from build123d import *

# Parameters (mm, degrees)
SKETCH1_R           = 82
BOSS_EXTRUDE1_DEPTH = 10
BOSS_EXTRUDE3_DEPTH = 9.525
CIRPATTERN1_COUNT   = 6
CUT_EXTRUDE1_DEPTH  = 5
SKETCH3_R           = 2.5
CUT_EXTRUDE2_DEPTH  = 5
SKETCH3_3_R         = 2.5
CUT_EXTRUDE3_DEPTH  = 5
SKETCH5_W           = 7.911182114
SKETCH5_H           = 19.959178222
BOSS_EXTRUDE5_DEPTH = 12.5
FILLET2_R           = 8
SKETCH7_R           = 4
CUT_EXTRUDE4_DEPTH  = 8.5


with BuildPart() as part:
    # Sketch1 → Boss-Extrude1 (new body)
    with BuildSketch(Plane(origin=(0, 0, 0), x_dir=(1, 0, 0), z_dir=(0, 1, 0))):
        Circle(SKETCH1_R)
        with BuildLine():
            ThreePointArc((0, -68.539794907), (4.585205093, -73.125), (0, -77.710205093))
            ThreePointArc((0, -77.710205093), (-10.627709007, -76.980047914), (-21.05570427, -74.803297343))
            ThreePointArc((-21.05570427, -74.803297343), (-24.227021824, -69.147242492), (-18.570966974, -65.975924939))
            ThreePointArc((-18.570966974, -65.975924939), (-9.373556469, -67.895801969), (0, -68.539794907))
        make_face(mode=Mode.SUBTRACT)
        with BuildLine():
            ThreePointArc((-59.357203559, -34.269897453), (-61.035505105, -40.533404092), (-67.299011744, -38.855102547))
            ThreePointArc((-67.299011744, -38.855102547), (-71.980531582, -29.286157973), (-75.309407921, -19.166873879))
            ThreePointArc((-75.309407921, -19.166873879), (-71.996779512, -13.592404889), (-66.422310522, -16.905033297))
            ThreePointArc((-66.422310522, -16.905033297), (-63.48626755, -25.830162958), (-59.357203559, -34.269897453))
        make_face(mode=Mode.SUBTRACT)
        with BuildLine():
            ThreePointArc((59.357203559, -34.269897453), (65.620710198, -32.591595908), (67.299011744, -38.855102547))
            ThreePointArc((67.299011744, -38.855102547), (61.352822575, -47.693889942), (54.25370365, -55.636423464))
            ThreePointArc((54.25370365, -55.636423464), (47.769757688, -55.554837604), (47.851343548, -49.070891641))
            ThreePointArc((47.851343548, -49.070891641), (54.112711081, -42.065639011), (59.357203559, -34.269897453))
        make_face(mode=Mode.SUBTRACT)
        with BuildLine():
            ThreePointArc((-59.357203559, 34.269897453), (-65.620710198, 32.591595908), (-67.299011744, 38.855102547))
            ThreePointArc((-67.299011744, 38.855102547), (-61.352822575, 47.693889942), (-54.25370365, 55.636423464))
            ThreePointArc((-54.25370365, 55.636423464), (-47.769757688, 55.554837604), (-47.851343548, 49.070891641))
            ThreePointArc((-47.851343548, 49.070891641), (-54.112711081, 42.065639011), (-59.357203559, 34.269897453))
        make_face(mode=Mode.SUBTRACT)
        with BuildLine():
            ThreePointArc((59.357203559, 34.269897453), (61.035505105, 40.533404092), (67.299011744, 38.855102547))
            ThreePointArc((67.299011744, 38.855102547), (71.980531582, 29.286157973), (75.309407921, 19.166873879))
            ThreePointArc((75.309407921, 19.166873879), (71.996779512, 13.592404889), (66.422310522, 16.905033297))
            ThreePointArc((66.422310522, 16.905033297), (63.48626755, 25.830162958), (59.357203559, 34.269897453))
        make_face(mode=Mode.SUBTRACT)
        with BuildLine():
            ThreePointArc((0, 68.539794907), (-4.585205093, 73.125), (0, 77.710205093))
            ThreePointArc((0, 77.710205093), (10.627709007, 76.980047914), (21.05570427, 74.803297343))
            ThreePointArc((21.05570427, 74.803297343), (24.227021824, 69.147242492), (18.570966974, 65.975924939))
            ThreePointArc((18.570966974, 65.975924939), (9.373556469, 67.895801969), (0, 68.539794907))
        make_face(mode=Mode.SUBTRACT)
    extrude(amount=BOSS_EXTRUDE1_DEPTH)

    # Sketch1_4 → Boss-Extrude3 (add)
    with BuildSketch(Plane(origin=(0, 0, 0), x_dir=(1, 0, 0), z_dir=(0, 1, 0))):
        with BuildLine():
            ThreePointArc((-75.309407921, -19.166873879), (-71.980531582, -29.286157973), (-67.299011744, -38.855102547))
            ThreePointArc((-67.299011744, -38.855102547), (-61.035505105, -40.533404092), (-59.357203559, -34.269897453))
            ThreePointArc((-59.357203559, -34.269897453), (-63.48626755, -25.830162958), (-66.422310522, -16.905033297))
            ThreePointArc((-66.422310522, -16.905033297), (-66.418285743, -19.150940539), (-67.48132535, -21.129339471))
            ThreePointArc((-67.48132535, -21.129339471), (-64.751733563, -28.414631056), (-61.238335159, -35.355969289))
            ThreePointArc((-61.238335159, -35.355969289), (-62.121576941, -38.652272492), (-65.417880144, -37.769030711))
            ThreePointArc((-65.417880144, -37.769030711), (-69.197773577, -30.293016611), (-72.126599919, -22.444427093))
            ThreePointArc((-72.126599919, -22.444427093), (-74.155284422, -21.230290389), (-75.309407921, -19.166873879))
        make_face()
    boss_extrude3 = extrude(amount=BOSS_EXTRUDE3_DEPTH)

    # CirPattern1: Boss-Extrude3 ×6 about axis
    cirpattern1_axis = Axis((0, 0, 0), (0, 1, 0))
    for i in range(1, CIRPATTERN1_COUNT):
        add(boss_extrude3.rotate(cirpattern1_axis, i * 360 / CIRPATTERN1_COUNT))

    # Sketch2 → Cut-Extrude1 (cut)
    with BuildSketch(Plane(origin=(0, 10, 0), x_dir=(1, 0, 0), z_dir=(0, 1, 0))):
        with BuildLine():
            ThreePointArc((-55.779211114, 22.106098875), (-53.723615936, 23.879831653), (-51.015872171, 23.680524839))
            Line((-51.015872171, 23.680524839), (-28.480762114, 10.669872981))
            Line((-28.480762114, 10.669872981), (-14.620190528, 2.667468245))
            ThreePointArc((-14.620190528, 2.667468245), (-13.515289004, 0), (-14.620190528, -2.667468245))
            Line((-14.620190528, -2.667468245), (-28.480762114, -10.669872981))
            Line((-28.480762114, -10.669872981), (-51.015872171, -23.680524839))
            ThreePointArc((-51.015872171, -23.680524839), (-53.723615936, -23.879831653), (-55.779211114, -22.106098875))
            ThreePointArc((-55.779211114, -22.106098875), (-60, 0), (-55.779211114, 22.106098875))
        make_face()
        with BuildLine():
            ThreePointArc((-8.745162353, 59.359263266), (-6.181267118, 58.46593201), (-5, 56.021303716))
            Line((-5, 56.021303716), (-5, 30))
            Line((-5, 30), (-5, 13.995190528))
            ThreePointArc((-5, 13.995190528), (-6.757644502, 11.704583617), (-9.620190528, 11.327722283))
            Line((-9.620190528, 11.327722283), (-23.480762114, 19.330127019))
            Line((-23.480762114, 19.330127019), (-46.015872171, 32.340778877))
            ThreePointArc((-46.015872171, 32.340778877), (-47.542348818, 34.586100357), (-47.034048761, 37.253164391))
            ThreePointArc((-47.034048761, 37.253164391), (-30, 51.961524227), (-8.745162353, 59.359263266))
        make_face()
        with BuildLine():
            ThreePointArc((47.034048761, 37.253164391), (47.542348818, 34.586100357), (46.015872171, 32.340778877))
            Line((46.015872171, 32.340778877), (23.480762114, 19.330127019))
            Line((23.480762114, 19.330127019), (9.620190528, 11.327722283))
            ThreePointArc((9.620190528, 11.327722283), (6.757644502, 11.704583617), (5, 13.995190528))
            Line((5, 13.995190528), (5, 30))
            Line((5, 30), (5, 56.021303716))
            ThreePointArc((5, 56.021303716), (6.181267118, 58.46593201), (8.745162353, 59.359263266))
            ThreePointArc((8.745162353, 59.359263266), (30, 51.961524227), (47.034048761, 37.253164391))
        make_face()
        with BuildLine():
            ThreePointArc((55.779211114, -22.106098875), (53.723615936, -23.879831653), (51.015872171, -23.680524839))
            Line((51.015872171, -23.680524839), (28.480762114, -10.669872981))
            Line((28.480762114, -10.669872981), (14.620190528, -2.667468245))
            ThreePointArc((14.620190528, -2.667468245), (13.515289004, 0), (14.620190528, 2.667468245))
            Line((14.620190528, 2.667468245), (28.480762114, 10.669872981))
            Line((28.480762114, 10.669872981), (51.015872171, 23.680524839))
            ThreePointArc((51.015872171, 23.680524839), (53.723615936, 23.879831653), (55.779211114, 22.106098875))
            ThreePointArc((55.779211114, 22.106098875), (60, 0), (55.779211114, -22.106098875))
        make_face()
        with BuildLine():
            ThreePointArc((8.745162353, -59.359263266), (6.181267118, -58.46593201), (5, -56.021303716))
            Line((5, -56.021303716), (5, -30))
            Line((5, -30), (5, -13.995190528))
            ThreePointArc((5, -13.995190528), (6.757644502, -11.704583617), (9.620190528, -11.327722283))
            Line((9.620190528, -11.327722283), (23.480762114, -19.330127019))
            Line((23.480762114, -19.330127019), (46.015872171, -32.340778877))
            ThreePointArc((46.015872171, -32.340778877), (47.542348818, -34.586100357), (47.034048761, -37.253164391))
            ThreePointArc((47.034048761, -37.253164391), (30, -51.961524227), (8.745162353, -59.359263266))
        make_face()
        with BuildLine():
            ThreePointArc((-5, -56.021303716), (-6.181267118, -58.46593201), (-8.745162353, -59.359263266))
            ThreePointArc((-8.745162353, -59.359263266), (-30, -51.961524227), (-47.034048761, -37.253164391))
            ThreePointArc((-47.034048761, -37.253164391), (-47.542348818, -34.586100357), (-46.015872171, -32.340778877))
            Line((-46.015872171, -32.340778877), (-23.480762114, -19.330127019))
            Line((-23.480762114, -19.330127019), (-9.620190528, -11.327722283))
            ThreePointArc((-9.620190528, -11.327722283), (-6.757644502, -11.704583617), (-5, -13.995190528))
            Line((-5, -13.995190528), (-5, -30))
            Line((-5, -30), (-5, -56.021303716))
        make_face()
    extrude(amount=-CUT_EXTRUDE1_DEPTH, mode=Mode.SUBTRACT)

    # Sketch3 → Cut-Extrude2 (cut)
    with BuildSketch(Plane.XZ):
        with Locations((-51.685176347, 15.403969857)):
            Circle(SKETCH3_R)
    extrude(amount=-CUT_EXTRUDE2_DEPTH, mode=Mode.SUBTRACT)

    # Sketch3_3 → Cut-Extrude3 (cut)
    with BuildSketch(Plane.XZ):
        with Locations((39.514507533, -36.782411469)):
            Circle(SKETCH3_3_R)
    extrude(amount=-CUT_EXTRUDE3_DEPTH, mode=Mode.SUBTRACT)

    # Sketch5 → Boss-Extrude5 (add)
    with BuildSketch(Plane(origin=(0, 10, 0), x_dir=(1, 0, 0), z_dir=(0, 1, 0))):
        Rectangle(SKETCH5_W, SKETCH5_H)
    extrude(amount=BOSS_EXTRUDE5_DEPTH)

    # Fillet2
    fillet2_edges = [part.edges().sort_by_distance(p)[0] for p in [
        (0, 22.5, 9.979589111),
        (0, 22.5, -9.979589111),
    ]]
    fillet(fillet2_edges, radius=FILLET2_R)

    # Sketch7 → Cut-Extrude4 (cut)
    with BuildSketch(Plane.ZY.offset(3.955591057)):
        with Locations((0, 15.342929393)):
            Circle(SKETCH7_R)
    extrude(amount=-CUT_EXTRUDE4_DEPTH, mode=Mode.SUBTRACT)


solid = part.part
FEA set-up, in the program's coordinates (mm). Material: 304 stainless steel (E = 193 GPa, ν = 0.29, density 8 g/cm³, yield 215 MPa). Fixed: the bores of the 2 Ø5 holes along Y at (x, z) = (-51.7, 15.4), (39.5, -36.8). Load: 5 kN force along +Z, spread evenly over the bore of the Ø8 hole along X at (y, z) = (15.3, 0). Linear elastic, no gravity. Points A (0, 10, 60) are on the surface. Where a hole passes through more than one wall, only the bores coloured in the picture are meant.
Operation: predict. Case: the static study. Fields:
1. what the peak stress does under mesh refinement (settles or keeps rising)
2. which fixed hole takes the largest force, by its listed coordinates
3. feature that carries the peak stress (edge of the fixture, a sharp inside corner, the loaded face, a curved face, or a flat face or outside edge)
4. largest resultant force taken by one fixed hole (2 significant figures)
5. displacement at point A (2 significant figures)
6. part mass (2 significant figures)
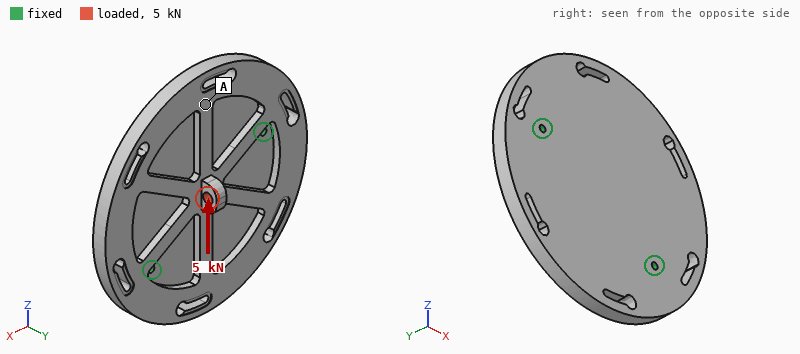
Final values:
keeps rising
(39.5, -36.8)
edge of the fixture
2.8 kN
0.15 mm
1.3 kg
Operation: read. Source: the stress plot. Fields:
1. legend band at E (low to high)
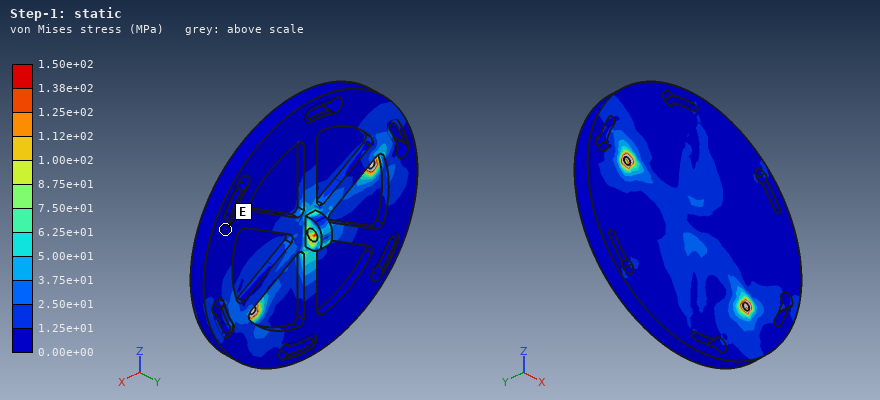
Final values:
0.00e+00 to 1.25e+01 MPa
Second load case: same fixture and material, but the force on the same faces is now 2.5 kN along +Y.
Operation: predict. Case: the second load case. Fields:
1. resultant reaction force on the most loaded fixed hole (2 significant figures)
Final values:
1.4 kN
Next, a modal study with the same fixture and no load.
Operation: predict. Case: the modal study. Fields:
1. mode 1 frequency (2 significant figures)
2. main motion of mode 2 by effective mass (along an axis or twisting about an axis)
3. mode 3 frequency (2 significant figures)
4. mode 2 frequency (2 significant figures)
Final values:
500 Hz
along Y
1500 Hz
1100 Hz
